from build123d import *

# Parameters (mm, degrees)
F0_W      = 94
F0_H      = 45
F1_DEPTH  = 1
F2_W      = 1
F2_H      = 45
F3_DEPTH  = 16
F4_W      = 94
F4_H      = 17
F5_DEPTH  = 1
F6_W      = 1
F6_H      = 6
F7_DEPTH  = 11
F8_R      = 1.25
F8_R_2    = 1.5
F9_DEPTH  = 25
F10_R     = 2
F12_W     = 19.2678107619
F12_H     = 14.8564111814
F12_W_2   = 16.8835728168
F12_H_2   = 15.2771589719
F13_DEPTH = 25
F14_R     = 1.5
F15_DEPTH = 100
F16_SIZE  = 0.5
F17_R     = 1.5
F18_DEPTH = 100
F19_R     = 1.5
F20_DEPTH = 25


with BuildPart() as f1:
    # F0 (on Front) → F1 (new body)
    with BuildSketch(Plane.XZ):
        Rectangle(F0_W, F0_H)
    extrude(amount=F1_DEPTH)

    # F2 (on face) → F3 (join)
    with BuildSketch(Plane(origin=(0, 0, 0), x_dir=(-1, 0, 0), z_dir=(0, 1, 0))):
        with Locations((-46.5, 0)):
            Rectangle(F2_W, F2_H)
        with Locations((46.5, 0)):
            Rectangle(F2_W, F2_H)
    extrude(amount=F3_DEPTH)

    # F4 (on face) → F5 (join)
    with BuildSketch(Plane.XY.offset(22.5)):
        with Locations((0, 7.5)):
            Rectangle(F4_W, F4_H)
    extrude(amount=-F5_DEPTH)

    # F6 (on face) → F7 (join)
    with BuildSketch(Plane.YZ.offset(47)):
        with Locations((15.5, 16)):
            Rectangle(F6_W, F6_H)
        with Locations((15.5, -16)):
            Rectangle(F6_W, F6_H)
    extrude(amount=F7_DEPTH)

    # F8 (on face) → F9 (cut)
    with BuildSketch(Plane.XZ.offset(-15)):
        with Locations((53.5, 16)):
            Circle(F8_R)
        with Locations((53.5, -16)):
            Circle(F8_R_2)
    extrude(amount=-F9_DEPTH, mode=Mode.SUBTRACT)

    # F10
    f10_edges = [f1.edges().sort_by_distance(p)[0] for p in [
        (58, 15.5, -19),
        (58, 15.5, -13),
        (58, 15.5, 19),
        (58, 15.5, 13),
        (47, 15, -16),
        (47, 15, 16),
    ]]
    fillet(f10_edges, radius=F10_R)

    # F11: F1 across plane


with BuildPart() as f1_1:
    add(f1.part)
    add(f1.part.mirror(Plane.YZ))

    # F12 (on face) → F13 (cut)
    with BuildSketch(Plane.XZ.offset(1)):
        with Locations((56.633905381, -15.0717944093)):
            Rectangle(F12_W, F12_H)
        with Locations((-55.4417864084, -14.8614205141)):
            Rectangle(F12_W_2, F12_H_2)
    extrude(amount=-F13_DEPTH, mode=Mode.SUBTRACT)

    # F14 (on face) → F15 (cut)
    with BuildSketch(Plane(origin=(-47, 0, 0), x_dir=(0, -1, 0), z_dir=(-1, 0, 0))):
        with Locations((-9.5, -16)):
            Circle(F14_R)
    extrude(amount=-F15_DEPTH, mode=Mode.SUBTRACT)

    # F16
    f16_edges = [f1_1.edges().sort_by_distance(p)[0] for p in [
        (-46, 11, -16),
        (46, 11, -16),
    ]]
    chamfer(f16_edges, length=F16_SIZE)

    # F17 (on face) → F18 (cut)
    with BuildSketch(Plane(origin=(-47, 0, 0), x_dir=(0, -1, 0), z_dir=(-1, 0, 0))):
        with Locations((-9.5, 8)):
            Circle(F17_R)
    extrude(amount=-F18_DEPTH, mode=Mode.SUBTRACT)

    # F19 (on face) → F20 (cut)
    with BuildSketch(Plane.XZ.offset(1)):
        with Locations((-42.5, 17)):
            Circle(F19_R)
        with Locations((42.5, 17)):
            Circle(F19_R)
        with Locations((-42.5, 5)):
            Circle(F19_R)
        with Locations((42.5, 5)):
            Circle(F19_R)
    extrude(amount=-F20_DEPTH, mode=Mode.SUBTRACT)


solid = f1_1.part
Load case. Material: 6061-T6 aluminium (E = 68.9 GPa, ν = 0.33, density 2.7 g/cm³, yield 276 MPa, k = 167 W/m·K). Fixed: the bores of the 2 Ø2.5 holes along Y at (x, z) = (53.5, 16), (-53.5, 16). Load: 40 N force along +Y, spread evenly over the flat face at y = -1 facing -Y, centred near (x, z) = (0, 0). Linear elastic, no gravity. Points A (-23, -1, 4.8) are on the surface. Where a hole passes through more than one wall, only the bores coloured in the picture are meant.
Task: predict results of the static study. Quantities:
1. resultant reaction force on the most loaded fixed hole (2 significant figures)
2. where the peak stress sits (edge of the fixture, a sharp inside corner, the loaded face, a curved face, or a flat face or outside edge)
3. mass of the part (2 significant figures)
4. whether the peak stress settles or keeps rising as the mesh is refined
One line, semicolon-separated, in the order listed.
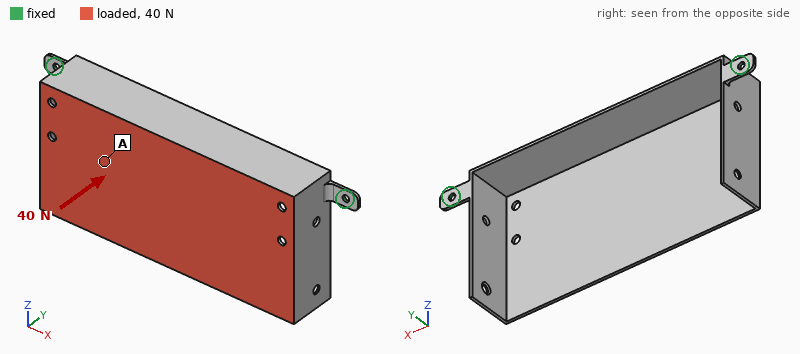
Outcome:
21 N; edge of the fixture; 19 g; keeps rising
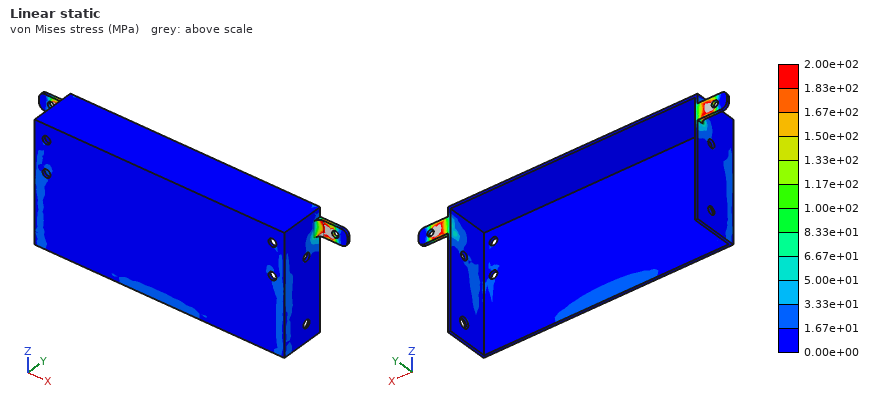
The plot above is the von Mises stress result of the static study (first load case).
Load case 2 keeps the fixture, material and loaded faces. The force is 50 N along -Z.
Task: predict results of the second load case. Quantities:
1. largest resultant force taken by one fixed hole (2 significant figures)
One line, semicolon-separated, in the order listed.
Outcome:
25 N
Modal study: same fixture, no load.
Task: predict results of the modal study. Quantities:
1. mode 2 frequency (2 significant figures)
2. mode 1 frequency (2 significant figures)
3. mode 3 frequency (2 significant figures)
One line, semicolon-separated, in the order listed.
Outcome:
480 Hz; 250 Hz; 750 Hz
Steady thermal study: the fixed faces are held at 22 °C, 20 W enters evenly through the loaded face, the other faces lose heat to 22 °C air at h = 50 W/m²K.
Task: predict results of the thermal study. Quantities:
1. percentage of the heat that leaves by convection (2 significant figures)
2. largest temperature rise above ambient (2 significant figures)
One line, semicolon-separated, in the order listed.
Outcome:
75 %; 40 K
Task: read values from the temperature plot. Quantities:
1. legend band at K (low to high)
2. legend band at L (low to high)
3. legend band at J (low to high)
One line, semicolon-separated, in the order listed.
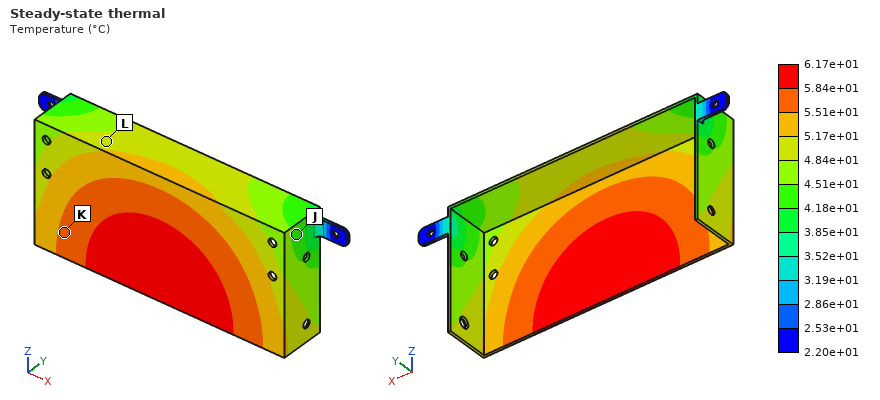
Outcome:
5.51e+01 to 5.84e+01 °C; 4.84e+01 to 5.17e+01 °C; 4.18e+01 to 4.51e+01 °C
